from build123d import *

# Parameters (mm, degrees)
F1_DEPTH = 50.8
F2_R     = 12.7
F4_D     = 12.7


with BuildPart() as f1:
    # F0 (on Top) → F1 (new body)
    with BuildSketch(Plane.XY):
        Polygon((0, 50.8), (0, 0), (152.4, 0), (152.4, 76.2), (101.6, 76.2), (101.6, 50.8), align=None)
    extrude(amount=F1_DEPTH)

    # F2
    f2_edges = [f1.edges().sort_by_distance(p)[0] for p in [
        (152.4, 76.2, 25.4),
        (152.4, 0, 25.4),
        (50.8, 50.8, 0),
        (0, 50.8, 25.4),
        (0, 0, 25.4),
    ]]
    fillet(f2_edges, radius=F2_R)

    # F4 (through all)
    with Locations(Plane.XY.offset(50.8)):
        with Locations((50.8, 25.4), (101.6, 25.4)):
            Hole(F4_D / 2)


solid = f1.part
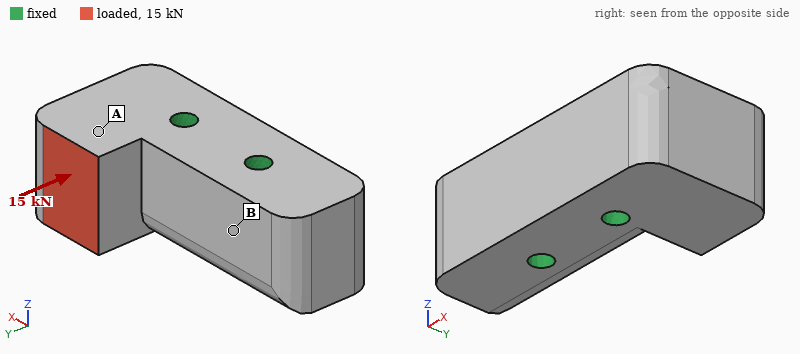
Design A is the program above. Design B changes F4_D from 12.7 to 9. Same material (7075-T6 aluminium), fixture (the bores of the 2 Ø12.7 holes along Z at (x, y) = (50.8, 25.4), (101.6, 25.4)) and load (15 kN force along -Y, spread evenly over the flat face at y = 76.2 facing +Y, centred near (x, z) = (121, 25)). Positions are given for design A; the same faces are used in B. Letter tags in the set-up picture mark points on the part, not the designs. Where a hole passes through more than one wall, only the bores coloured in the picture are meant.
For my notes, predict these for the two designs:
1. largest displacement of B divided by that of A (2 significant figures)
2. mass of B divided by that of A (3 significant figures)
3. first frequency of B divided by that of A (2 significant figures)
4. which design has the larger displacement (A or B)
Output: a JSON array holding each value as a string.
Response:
["1.2", "1.01", "0.92", "B"]
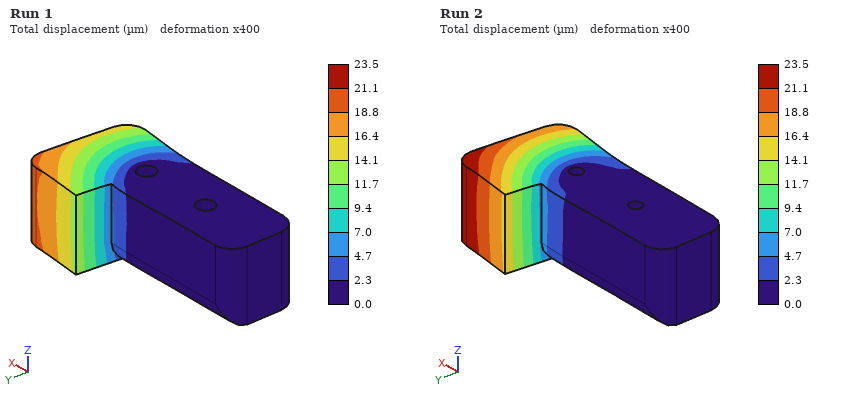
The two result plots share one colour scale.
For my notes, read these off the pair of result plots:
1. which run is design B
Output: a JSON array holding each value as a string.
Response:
["Run 2"]
